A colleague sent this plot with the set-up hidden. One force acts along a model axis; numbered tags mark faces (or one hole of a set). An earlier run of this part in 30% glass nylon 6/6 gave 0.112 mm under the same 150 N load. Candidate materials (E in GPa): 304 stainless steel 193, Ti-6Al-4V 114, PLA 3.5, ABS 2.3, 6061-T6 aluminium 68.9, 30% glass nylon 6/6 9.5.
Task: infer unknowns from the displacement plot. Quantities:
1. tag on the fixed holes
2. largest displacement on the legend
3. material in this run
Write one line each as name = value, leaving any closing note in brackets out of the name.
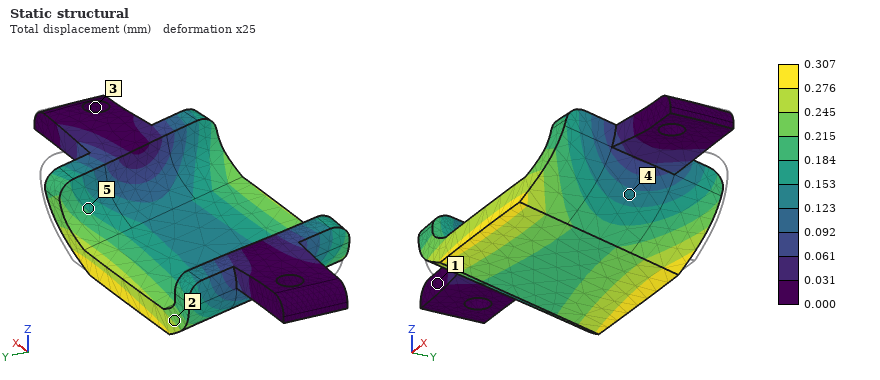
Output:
tag on the fixed holes = 3
largest displacement on the legend = 0.307 mm
material in this run = PLA
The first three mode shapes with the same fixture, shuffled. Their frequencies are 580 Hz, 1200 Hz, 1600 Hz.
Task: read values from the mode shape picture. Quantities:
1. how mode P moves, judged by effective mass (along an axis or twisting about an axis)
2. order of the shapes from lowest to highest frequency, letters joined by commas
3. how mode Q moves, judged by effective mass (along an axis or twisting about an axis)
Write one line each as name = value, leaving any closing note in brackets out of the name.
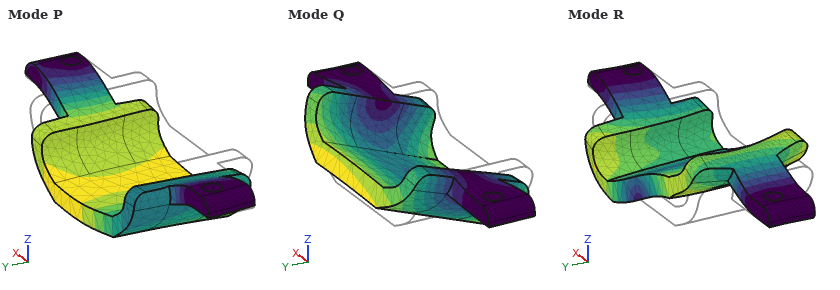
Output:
how mode P moves, judged by effective mass = along Z
order of the shapes from lowest to highest frequency, letters joined by commas = Q, P, R
how mode Q moves, judged by effective mass = along Y
